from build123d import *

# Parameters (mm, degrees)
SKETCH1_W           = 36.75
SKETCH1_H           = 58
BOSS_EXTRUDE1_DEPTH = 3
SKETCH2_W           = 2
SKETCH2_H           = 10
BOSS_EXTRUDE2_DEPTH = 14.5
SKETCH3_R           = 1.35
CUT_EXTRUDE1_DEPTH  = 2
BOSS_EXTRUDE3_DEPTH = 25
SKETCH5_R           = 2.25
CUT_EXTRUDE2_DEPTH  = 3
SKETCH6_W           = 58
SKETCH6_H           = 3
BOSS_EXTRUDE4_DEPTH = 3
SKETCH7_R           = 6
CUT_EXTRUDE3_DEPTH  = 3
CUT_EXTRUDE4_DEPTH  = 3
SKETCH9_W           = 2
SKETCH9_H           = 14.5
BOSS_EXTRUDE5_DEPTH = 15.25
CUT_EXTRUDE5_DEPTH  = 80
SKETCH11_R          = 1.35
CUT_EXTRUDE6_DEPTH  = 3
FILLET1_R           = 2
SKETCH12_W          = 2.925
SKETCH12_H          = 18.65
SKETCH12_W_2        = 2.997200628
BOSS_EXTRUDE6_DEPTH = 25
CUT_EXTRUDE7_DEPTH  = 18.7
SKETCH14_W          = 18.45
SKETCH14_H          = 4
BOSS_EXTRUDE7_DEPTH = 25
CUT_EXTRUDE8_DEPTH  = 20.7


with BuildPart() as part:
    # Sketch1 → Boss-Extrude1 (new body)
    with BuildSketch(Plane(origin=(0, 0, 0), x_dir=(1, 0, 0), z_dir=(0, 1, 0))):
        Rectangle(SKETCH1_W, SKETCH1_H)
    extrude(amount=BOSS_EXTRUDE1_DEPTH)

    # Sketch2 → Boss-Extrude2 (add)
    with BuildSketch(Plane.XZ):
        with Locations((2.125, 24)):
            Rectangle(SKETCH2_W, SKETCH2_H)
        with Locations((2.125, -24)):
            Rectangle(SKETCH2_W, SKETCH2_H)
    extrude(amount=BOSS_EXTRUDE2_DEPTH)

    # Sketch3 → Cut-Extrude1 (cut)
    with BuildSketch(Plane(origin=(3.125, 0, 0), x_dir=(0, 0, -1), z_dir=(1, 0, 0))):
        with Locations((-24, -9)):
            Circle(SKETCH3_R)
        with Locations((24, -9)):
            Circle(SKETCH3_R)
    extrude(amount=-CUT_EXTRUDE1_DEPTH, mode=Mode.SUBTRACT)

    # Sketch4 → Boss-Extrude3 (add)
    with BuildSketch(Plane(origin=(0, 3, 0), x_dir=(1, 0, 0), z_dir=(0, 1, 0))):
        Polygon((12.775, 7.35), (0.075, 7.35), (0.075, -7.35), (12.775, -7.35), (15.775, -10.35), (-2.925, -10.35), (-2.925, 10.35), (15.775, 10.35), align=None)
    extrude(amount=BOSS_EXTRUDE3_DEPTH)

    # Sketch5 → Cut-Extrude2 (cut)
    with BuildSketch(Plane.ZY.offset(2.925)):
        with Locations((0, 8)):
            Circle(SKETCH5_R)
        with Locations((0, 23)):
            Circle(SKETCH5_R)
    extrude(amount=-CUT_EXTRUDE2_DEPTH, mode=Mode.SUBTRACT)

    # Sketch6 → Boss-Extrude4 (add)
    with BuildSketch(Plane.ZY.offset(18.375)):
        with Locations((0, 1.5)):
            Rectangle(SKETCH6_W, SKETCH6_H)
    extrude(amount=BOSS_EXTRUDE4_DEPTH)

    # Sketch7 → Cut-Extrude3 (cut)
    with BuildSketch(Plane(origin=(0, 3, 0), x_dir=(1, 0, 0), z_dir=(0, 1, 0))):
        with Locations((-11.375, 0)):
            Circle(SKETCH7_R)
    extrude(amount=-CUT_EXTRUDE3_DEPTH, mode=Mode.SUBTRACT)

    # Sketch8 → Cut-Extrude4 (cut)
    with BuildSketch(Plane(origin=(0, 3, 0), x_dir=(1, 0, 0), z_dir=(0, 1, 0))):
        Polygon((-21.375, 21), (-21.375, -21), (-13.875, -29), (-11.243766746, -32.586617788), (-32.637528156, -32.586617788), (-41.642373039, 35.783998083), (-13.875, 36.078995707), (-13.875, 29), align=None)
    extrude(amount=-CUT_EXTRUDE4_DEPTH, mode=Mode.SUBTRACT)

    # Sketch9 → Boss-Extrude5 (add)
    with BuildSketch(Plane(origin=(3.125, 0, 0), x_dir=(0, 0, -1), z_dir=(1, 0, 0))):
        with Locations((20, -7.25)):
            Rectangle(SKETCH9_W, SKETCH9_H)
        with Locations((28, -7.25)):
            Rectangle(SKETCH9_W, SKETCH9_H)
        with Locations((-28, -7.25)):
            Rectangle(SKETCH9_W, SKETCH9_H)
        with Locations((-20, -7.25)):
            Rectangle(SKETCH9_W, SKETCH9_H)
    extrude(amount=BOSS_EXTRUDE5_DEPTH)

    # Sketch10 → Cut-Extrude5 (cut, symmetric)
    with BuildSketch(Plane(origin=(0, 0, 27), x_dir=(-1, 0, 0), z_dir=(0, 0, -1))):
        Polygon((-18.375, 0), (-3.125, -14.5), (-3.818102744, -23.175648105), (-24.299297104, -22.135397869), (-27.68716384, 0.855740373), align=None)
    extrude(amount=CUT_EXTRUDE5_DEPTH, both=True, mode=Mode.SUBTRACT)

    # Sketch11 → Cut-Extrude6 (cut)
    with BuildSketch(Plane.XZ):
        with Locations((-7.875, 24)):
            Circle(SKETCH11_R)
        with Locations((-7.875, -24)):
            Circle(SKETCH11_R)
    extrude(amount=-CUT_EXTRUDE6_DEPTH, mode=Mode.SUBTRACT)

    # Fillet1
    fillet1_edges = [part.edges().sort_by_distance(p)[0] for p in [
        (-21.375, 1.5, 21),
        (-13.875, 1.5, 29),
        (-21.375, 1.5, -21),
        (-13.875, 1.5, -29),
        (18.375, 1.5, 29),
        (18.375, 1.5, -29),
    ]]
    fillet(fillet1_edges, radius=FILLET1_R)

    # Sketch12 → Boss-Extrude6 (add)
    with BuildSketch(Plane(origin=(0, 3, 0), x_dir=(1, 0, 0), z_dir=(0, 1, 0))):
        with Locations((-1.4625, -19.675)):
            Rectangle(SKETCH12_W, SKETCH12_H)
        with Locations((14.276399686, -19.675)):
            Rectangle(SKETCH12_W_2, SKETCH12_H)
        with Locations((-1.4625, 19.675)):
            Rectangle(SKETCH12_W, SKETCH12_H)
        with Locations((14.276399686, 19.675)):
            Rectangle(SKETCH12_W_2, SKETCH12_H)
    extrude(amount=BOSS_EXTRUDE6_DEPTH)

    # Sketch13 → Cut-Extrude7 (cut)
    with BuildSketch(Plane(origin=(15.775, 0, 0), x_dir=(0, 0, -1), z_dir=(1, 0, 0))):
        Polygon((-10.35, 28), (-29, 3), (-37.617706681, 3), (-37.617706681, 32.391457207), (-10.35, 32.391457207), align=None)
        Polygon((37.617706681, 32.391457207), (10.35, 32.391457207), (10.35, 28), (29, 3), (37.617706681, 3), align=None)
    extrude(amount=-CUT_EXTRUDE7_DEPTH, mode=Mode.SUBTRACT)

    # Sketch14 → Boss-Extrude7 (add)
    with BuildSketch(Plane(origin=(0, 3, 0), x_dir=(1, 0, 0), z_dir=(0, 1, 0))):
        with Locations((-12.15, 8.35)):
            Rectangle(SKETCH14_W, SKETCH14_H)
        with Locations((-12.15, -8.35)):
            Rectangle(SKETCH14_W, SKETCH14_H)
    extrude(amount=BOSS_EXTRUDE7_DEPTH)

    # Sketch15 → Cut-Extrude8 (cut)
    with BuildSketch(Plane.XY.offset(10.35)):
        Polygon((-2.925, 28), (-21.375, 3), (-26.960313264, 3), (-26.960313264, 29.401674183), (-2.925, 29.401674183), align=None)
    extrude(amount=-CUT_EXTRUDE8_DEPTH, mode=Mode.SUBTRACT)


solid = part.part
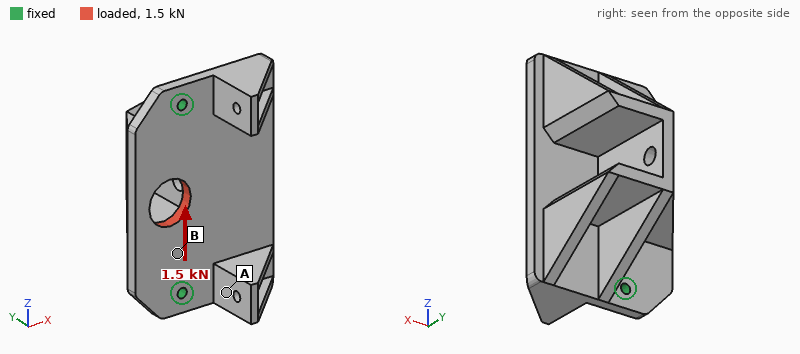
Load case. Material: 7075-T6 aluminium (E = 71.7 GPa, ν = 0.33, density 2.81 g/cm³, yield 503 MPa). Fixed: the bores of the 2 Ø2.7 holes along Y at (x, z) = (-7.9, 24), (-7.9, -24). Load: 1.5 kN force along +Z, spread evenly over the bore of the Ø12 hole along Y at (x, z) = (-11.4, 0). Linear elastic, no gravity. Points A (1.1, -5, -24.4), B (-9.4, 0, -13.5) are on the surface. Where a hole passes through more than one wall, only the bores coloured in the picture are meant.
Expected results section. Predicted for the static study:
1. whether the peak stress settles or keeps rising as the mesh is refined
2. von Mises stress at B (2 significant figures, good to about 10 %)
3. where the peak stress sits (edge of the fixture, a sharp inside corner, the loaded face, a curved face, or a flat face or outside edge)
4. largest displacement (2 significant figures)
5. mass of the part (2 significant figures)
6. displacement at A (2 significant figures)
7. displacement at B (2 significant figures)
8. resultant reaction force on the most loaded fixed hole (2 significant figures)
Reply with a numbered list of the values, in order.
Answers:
1. keeps rising
2. 17 MPa
3. edge of the fixture
4. 7.0 µm
5. 45 g
6. 2.1 µm
7. 3.1 µm
8. 760 N
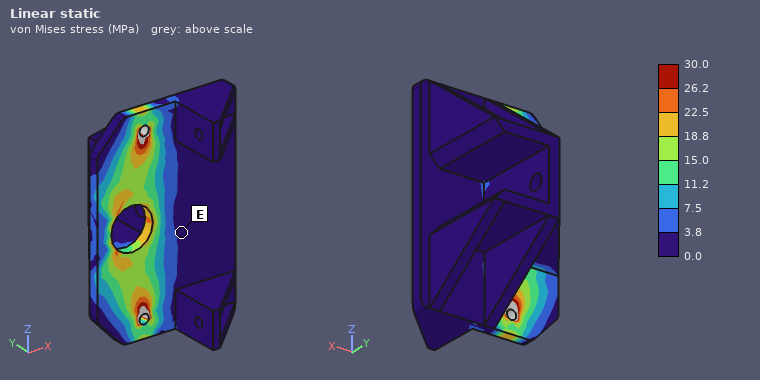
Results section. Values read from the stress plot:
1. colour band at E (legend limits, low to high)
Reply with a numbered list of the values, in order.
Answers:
1. 0.0 to 3.8 MPa
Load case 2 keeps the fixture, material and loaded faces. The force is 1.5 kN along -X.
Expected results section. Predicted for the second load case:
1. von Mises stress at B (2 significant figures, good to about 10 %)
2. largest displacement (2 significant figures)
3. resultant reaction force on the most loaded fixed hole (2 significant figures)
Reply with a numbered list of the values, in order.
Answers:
1. 15 MPa
2. 15 µm
3. 760 N
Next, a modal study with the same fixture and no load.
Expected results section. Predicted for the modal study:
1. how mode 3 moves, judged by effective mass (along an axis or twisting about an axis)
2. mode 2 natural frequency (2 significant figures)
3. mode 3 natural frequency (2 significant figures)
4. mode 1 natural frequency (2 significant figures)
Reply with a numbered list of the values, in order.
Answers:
1. along Y
2. 5400 Hz
3. 6800 Hz
4. 1600 Hz
